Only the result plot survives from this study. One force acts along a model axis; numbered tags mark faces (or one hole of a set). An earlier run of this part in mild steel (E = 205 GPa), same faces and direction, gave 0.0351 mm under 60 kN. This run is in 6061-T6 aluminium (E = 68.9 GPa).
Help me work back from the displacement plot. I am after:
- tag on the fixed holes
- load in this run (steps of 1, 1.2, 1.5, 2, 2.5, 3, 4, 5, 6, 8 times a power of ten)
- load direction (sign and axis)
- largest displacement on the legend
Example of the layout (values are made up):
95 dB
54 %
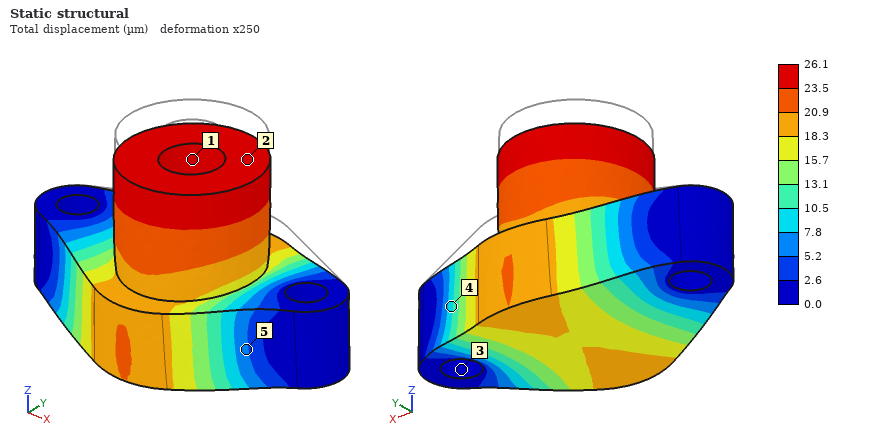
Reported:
3
15 kN
-Z
26.1 µm
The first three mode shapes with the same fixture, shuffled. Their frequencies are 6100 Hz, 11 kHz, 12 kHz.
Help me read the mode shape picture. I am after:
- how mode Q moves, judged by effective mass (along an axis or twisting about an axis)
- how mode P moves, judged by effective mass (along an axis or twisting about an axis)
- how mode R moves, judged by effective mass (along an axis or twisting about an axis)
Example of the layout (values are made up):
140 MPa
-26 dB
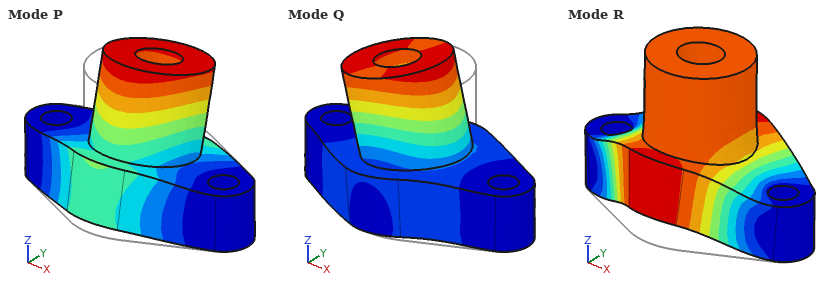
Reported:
along X
along Y
along Z
